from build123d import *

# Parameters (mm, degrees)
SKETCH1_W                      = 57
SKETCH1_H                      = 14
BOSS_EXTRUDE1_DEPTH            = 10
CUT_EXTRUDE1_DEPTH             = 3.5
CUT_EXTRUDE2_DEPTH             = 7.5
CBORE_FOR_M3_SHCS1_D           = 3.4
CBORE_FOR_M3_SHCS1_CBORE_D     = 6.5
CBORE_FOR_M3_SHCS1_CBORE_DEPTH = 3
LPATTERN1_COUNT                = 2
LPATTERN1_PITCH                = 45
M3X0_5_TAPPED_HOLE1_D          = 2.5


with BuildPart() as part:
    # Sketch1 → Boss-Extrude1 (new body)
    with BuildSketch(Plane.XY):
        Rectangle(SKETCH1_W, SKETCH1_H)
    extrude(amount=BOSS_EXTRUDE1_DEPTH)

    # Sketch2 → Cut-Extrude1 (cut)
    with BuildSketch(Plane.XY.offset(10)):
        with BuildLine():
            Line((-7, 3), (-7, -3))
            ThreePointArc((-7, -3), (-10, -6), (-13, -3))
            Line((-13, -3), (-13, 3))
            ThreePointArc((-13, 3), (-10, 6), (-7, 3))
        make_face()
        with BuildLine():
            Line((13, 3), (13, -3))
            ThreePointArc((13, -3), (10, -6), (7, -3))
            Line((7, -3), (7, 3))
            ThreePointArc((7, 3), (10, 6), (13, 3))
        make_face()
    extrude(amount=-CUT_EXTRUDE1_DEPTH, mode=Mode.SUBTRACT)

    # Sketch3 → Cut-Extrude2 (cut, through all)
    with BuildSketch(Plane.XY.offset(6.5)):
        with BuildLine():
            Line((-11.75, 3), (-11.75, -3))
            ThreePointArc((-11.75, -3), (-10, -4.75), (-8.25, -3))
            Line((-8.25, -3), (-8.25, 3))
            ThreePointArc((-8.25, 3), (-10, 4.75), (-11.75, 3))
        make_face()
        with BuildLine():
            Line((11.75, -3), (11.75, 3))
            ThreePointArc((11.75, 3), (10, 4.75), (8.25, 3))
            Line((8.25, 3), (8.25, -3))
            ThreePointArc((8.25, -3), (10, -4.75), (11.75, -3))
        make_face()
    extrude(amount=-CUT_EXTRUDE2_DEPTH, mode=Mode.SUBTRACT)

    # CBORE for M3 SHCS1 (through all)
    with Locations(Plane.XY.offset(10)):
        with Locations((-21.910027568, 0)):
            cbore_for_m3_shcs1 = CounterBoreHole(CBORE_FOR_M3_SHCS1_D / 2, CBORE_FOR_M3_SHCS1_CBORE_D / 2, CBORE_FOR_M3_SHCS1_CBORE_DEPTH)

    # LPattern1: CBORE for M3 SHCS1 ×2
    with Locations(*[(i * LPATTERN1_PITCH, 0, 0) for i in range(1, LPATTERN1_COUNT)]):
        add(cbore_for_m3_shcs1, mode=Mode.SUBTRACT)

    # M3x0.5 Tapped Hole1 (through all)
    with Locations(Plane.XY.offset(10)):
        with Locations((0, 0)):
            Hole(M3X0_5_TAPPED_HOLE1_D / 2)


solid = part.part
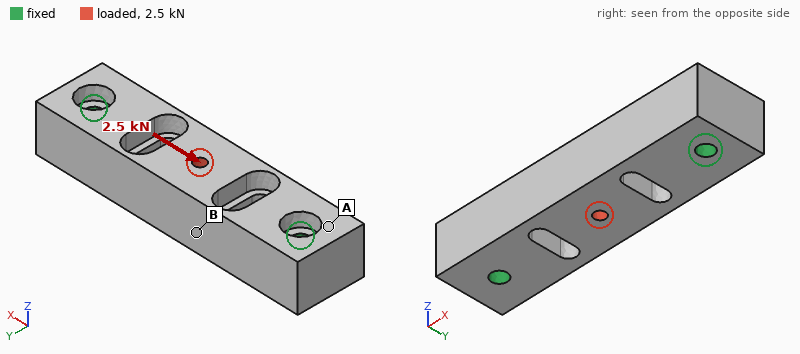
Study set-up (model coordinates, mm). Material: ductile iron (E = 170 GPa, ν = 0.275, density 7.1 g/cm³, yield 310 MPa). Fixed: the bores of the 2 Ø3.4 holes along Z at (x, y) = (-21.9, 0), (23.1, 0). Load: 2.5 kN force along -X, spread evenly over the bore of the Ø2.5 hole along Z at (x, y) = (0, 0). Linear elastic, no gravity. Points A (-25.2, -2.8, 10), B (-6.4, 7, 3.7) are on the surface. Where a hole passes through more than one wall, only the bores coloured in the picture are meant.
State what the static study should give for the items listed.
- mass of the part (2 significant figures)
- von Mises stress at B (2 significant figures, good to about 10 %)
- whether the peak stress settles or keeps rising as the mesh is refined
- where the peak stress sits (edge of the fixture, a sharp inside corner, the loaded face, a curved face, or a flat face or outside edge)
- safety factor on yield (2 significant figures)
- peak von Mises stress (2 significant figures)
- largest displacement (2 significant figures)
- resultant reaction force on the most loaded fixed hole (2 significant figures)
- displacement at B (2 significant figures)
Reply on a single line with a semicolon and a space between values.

48 g; 24 MPa; settles; a curved face; 3.4; 92 MPa; 3.8 µm; 1.3 kN; 2.1 µm
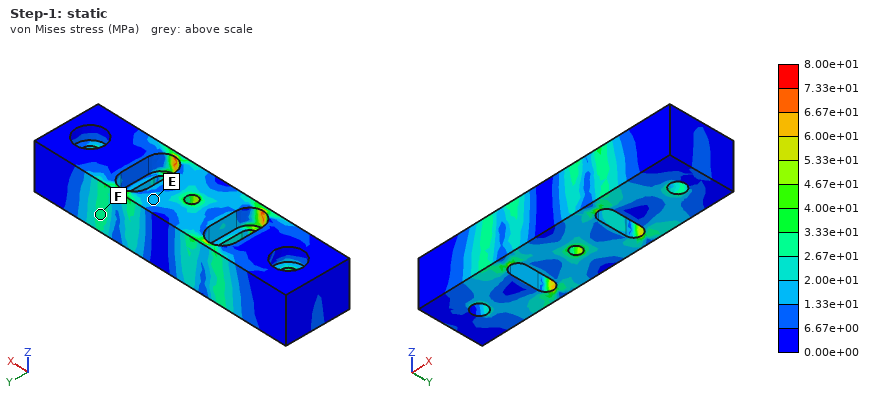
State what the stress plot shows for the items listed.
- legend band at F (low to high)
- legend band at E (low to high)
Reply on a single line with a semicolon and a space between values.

2.67e+01 to 3.33e+01 MPa; 1.33e+01 to 2.00e+01 MPa
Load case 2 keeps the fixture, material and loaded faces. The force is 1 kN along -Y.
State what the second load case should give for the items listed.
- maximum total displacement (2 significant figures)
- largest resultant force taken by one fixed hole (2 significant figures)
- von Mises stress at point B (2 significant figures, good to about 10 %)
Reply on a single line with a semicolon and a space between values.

8.6 µm; 510 N; 40 MPa
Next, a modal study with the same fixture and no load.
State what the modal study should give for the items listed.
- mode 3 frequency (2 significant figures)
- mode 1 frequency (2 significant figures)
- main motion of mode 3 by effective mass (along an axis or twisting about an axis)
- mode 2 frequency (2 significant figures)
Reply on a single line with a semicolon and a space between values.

22 kHz; 14 kHz; twisting about X; 15 kHz
